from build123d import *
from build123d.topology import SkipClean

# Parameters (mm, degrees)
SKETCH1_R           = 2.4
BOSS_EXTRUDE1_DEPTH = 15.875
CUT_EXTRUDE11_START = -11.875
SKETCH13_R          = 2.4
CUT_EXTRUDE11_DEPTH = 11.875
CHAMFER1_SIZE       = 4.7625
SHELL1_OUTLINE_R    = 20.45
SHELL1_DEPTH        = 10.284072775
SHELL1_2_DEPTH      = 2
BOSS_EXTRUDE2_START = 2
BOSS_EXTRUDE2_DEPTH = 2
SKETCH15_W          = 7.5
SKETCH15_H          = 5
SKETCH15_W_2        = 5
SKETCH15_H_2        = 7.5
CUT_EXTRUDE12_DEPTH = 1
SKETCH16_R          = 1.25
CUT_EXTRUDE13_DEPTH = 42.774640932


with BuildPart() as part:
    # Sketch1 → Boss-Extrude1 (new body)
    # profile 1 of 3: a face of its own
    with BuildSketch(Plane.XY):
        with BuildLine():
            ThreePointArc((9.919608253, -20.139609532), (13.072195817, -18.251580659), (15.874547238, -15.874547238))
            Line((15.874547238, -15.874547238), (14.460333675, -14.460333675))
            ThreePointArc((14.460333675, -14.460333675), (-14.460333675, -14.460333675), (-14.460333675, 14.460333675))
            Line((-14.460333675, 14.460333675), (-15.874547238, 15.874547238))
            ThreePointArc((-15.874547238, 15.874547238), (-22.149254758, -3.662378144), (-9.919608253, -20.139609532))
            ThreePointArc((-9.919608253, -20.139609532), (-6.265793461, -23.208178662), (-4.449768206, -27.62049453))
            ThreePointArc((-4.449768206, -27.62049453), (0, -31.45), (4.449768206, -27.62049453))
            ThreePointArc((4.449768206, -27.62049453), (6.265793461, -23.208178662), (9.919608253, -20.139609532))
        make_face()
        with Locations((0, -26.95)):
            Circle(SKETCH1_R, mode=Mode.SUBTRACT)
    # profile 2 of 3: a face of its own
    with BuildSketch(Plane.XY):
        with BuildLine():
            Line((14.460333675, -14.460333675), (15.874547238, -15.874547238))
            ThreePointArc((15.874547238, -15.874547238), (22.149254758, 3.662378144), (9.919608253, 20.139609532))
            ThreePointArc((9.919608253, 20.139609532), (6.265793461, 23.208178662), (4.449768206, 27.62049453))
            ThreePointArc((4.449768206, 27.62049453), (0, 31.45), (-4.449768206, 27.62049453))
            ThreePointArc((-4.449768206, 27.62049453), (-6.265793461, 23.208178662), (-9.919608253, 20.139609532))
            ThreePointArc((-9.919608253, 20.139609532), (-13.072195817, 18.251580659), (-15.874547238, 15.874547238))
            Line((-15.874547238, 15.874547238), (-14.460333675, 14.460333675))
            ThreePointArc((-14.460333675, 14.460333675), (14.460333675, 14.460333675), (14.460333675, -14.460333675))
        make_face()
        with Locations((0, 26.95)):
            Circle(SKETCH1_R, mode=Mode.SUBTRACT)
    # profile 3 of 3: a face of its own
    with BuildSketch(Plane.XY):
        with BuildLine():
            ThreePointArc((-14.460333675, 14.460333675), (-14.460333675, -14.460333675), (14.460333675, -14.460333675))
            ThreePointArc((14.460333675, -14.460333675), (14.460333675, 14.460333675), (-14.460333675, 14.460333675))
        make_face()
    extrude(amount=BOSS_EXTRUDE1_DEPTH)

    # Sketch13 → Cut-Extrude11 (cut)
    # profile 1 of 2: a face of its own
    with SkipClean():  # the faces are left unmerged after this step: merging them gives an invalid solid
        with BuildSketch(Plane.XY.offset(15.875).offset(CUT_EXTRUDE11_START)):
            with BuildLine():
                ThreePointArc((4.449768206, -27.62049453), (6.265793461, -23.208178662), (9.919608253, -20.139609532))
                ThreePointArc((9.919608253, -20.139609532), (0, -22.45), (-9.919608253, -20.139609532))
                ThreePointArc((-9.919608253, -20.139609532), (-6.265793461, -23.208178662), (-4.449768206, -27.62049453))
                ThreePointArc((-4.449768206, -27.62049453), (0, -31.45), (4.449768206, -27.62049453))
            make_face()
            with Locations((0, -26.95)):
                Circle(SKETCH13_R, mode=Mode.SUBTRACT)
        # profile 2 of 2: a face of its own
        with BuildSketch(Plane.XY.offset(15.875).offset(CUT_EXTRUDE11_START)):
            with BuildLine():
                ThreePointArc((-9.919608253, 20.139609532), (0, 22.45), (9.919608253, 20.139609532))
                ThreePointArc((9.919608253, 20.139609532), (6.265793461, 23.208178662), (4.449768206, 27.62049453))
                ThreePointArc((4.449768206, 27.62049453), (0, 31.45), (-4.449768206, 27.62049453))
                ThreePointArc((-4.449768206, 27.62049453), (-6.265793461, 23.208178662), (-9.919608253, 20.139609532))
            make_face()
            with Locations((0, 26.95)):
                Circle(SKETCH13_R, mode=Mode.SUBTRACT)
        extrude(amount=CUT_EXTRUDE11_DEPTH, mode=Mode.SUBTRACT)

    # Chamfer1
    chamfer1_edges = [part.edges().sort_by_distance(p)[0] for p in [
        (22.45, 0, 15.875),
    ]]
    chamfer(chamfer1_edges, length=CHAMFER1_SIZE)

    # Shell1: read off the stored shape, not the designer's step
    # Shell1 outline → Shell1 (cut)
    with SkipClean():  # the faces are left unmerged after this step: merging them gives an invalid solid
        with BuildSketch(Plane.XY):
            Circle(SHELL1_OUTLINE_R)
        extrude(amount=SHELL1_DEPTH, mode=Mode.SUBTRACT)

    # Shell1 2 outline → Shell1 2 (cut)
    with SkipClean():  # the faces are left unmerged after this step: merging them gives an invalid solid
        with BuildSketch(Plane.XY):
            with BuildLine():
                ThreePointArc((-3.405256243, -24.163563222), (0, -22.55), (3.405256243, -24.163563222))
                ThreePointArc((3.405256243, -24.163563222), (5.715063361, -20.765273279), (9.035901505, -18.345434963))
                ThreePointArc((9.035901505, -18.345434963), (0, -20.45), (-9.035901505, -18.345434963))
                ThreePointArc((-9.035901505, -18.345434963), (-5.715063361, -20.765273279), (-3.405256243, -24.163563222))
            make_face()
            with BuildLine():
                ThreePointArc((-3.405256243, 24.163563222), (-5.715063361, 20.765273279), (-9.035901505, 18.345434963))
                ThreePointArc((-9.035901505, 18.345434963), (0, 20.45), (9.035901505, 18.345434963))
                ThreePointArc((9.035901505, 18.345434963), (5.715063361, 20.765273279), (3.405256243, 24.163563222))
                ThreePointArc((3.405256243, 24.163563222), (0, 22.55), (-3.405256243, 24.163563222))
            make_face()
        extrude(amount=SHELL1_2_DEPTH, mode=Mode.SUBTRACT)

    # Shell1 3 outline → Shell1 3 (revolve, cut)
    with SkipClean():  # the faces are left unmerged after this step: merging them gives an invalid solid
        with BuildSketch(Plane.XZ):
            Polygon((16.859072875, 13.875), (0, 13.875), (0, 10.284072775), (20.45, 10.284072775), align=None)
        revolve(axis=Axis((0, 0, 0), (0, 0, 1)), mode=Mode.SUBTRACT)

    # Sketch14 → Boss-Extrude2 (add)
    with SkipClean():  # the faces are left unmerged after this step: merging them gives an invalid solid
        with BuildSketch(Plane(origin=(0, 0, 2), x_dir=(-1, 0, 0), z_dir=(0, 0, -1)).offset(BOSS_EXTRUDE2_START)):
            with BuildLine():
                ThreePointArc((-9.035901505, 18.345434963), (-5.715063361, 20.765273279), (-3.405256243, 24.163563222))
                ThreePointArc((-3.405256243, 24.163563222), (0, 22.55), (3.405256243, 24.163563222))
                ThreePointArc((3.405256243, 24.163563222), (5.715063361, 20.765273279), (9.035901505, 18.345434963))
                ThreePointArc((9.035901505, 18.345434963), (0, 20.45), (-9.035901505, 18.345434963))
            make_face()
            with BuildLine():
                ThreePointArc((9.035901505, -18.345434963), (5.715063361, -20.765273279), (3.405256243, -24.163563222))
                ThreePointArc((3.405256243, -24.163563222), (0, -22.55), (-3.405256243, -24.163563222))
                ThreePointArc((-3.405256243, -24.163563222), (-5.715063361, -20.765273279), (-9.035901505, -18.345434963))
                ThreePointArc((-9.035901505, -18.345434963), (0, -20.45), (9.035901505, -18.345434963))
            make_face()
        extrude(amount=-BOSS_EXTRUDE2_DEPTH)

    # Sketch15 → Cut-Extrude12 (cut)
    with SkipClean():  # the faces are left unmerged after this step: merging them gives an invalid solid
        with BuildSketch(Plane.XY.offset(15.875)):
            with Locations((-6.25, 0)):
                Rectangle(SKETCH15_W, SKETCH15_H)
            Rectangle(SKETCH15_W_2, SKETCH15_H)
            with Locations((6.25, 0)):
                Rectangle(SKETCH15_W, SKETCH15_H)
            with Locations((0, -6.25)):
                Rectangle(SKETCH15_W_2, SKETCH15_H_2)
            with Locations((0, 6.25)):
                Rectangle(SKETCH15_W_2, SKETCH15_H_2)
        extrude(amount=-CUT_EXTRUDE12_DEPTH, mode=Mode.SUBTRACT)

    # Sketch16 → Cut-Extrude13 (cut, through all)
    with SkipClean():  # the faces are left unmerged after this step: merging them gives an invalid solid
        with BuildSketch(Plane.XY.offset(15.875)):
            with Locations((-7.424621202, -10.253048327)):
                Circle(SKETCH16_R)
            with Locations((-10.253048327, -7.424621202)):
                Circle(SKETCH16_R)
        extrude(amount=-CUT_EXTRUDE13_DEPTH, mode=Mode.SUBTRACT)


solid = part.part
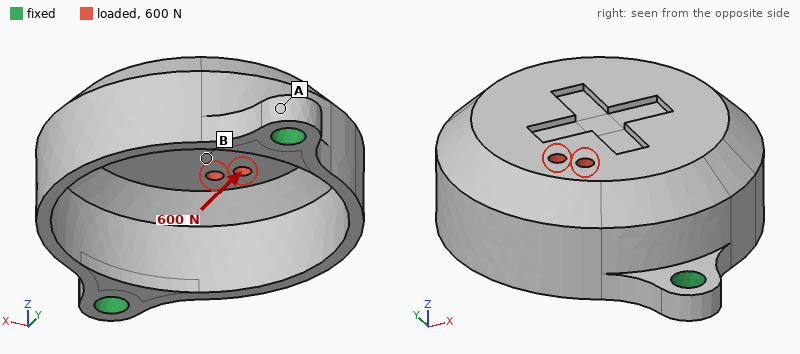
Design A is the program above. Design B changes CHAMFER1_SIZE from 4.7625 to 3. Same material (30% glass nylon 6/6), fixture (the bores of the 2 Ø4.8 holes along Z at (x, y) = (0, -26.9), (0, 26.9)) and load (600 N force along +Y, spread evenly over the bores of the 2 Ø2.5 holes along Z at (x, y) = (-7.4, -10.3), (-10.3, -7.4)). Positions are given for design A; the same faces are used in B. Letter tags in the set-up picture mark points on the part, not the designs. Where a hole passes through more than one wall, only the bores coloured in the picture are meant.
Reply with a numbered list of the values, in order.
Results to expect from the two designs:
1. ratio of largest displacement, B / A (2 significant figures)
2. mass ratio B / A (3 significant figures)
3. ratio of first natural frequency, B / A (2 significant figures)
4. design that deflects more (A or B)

1. 0.89
2. 1.13
3. 0.92
4. A
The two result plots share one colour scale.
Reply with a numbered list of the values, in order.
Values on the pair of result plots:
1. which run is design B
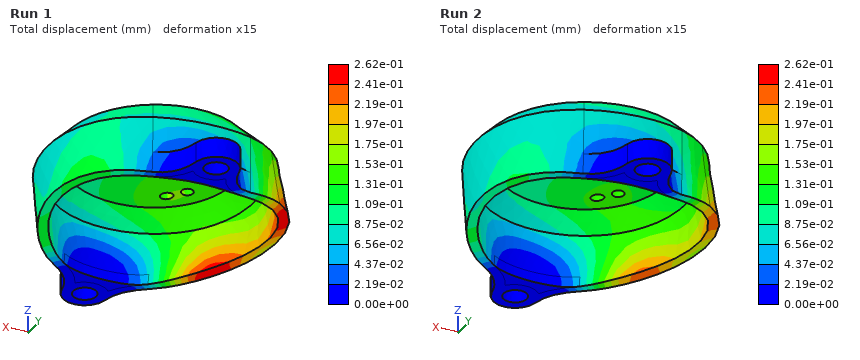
1. Run 2
